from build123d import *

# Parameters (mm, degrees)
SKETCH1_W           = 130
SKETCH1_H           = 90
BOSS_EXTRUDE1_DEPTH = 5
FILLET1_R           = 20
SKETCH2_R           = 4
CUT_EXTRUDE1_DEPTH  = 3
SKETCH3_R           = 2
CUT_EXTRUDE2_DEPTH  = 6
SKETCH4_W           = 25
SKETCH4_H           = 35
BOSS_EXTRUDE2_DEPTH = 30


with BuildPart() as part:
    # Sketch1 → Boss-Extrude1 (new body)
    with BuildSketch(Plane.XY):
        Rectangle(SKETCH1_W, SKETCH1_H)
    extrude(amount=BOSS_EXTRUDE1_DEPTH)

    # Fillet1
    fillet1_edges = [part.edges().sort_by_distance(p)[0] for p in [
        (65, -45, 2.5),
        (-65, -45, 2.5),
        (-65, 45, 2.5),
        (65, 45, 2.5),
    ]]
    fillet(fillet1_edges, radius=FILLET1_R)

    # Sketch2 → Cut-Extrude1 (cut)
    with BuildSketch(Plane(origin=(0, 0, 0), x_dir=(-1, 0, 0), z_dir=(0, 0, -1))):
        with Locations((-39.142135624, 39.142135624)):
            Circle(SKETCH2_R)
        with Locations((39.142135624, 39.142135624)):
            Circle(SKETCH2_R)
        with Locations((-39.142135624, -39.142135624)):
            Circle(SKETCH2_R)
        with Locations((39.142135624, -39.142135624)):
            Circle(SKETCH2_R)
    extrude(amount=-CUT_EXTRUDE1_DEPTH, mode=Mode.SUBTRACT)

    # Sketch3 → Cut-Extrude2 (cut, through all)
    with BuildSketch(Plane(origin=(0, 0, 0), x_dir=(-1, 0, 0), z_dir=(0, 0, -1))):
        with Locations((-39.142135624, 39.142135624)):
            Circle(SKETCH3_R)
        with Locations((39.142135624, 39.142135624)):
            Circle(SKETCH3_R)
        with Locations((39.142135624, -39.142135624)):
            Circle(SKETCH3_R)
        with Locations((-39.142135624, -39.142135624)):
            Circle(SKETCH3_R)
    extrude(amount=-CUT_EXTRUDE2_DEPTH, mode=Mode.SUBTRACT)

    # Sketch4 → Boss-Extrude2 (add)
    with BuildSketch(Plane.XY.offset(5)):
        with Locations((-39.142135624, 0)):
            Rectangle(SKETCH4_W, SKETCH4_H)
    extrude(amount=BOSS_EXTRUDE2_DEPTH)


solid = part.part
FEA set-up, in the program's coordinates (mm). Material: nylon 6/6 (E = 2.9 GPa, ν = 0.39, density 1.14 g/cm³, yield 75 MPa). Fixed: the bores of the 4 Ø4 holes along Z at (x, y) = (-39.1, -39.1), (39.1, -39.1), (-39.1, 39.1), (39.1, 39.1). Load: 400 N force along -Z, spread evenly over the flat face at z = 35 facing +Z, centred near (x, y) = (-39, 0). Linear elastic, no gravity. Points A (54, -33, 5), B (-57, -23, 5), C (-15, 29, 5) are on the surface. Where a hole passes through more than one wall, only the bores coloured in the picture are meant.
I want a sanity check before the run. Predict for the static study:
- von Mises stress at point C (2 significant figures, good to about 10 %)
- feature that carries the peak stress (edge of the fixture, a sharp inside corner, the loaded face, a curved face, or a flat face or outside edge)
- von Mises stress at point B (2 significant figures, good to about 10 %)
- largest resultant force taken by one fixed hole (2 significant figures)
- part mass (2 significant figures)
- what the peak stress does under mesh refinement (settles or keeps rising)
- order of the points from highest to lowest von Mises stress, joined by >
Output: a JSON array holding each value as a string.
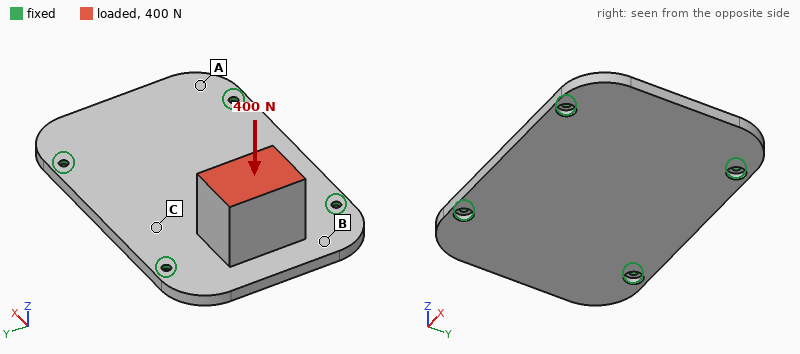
["3.3 MPa", "edge of the fixture", "5.8 MPa", "280 N", "94 g", "keeps rising", "B > C > A"]
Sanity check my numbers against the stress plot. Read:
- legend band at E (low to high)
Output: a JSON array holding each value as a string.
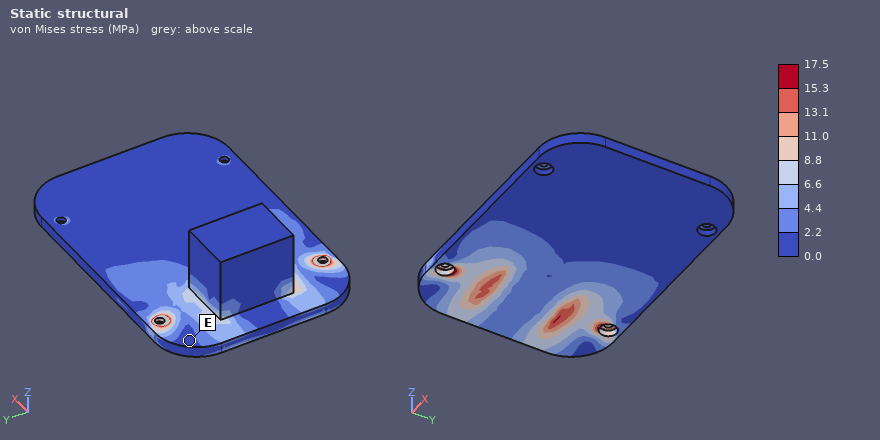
["0.0 to 2.2 MPa"]
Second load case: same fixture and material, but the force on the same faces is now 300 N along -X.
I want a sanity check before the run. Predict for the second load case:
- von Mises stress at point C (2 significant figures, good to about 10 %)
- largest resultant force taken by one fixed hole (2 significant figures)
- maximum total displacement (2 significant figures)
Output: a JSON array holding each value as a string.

["7.9 MPa", "300 N", "1.7 mm"]
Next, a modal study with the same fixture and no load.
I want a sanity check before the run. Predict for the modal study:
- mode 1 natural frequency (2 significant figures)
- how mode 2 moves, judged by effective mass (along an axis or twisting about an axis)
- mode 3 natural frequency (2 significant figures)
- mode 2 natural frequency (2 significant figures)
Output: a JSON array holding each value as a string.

["510 Hz", "along Z", "770 Hz", "660 Hz"]
